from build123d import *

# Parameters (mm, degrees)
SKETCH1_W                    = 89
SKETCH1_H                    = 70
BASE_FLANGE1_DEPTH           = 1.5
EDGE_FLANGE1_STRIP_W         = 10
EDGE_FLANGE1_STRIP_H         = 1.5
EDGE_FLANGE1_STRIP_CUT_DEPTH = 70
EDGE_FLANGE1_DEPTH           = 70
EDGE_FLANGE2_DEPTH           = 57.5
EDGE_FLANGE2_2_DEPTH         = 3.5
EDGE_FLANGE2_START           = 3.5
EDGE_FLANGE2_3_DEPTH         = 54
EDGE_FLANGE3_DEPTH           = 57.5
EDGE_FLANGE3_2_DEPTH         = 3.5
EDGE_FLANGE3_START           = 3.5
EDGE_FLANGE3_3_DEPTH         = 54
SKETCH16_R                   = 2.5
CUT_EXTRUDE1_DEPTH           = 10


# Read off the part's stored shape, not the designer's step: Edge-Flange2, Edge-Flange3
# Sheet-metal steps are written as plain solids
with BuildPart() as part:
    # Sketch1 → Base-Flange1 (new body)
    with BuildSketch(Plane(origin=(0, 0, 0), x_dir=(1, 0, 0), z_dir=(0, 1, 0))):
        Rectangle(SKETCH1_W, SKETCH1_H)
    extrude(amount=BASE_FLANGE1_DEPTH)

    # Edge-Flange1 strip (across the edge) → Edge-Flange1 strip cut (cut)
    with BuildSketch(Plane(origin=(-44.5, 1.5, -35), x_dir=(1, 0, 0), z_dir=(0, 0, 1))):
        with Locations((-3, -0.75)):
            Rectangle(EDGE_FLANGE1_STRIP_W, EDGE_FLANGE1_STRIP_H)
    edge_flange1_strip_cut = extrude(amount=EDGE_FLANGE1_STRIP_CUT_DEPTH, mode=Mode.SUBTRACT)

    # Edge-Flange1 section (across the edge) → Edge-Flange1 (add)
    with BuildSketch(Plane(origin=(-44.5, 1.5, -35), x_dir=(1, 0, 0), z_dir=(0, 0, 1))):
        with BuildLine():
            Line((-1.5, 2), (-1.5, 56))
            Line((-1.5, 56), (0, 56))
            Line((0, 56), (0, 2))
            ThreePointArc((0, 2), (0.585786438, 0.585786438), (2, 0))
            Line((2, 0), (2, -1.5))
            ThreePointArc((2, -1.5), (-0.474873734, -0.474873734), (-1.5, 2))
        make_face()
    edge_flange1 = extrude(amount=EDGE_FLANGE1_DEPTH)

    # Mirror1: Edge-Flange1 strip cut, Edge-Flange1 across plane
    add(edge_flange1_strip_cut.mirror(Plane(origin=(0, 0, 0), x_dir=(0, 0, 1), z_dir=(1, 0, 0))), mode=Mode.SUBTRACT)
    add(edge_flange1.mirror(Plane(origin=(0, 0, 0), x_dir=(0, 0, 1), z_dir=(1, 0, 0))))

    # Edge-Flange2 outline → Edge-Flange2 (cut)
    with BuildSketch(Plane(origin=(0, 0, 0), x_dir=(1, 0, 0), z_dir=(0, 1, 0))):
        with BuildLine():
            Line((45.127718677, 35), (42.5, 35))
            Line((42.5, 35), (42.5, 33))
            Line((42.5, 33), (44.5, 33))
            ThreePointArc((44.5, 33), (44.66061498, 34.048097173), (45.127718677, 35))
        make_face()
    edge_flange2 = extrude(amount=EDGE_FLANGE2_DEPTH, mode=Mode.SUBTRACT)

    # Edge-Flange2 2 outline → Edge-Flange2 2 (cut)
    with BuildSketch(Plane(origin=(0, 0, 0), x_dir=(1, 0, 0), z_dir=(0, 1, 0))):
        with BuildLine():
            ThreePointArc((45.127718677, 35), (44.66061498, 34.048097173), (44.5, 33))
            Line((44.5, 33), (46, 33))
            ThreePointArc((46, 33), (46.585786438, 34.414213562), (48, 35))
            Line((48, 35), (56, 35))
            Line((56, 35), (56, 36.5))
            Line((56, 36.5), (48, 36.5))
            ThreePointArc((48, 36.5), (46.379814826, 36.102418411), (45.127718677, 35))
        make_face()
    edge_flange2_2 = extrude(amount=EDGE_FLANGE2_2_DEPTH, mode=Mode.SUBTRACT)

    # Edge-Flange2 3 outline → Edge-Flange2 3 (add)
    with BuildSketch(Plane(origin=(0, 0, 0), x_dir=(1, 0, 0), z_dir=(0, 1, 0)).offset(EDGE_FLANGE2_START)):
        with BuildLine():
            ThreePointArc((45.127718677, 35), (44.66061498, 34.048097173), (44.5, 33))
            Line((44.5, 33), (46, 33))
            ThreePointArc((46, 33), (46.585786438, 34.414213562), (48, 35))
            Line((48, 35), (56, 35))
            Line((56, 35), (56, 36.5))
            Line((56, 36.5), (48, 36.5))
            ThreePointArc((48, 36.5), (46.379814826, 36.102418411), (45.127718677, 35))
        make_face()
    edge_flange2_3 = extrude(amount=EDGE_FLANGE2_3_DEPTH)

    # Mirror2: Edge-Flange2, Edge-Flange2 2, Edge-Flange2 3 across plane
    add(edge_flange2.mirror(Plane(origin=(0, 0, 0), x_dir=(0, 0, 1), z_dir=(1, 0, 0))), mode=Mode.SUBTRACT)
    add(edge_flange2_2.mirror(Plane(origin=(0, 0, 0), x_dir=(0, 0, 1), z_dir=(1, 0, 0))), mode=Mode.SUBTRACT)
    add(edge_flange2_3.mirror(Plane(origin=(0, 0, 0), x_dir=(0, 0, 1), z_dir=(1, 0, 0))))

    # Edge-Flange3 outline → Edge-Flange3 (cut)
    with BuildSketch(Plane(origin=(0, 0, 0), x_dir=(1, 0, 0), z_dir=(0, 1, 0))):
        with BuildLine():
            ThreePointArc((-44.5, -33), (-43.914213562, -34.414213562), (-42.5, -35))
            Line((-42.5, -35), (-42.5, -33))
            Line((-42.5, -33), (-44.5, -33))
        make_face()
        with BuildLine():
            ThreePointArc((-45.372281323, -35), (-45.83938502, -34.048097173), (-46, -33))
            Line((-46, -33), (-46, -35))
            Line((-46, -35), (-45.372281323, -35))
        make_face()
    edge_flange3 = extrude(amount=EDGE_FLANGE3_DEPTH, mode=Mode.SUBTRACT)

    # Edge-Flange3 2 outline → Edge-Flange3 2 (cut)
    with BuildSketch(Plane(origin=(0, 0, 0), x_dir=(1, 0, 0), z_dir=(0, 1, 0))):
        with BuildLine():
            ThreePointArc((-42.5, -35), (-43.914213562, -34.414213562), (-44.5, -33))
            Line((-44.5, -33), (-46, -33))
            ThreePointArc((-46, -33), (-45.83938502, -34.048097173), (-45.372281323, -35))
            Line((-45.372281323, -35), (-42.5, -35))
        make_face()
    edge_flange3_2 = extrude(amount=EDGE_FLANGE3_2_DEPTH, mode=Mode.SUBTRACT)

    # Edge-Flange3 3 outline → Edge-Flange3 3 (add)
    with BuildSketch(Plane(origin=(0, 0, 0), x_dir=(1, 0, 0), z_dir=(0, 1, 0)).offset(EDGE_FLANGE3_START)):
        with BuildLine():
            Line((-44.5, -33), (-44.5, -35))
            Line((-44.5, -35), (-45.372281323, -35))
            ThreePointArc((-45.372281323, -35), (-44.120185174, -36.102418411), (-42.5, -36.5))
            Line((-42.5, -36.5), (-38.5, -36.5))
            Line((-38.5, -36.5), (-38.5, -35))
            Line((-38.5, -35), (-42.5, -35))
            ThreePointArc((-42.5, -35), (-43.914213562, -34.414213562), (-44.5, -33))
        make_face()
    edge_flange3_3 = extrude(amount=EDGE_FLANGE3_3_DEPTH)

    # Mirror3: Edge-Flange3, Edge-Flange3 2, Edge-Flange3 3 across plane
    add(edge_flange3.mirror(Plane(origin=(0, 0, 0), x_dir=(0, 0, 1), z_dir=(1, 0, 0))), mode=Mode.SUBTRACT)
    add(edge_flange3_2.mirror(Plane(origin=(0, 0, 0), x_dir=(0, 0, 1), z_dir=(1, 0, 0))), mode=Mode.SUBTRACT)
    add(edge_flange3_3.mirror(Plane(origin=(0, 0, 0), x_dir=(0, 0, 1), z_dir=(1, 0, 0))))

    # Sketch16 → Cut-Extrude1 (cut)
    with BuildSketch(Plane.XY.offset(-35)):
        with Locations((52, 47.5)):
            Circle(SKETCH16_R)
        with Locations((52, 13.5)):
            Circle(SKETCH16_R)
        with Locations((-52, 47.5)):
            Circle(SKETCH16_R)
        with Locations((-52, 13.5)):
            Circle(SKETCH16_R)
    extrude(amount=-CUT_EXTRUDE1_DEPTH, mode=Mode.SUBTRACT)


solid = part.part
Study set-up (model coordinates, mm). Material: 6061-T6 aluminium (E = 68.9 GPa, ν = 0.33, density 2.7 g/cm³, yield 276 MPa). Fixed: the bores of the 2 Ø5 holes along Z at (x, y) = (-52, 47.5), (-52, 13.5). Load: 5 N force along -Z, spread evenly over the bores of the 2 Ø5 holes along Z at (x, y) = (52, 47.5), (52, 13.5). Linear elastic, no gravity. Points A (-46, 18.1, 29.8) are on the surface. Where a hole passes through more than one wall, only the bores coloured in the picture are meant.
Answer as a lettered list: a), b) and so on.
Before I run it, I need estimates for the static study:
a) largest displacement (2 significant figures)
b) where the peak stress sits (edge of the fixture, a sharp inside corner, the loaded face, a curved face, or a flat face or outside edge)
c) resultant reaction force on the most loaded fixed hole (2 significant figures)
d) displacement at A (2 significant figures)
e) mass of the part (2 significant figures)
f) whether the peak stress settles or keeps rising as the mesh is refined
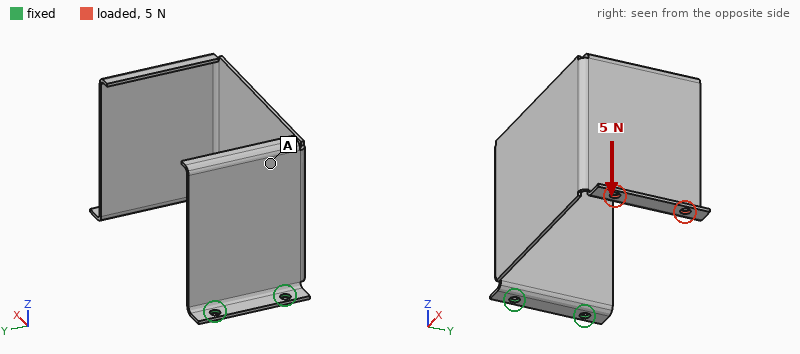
a) 1.6 mm
b) a sharp inside corner
c) 9.2 N
d) 0.61 mm
e) 64 g
f) keeps rising
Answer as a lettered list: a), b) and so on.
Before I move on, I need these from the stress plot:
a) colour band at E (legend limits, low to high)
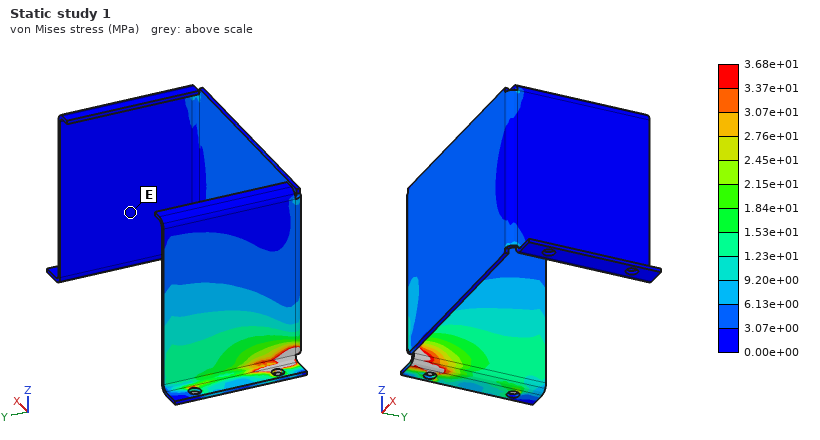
a) 0.00e+00 to 3.07e+00 MPa
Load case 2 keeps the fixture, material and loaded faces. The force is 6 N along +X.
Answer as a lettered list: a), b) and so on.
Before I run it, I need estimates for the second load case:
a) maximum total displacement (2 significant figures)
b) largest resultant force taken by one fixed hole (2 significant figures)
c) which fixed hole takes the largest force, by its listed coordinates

a) 1.3 mm
b) 3.2 N
c) (-52, 13.5)
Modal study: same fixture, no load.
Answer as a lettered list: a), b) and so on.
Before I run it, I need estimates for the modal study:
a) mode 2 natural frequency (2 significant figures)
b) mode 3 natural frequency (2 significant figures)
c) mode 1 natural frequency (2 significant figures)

a) 62 Hz
b) 160 Hz
c) 50 Hz
